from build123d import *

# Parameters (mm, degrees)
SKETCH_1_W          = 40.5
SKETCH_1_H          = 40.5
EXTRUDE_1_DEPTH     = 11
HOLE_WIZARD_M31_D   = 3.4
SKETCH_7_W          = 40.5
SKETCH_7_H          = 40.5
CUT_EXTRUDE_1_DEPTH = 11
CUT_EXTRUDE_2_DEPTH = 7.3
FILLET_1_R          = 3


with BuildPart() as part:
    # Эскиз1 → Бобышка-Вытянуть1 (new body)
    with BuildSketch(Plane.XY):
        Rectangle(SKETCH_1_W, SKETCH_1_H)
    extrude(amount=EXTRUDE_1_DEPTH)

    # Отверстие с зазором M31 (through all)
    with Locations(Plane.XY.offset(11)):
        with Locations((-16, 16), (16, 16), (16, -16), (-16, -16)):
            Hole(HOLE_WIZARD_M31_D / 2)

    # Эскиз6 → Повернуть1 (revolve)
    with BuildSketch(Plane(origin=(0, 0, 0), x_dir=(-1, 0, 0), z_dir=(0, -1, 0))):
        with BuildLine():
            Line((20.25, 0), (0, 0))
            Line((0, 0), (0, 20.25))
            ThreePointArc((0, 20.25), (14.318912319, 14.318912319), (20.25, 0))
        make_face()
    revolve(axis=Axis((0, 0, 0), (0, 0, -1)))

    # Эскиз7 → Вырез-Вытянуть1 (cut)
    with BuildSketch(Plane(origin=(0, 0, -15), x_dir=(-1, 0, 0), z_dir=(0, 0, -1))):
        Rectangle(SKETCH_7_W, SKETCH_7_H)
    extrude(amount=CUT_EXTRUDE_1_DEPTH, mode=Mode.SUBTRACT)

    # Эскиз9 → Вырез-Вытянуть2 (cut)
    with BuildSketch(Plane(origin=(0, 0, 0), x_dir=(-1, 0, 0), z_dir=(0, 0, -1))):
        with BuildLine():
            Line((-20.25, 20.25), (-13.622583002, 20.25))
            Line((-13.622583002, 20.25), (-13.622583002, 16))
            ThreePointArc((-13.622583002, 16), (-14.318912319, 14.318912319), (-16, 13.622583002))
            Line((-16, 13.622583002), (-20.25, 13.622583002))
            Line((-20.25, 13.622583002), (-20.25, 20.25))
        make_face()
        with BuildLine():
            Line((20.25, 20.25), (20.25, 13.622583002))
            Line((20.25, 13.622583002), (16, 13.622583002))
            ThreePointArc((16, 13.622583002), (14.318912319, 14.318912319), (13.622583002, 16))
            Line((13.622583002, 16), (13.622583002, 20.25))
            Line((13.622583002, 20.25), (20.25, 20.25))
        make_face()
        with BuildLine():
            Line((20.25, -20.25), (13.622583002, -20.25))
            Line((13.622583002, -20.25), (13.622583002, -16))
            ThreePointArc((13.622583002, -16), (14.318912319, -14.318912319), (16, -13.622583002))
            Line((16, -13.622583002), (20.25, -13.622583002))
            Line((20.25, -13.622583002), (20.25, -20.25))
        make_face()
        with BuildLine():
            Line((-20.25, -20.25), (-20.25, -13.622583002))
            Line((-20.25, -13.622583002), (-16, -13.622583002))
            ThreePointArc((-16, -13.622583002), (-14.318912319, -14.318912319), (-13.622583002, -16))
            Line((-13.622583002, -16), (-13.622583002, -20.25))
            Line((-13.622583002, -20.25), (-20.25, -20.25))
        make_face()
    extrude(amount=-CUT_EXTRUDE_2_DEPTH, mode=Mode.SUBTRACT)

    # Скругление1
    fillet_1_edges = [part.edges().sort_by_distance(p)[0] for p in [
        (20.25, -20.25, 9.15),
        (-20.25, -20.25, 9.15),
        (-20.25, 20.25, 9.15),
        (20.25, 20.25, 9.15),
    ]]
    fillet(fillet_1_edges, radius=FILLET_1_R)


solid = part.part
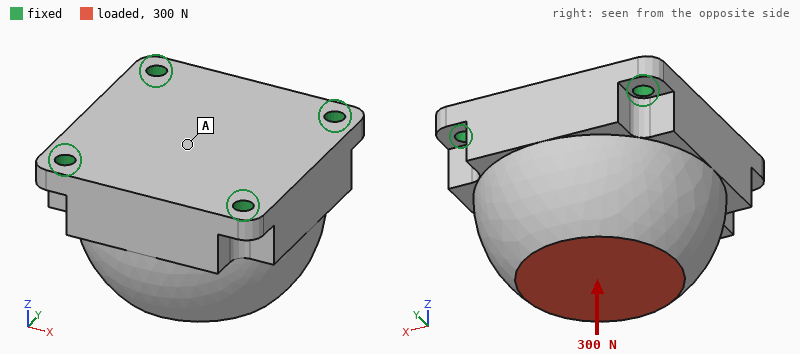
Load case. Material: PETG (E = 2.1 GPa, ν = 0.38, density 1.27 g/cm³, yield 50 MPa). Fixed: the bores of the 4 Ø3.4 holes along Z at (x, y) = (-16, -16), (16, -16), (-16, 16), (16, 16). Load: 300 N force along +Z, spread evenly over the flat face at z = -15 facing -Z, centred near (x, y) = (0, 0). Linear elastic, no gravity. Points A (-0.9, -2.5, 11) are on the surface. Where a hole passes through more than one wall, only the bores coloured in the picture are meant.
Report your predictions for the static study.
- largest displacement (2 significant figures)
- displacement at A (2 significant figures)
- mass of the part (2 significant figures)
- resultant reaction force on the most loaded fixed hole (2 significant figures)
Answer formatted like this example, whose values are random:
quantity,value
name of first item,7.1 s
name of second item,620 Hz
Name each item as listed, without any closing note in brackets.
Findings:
quantity,value
largest displacement,15 µm
displacement at A,12 µm
mass of the part,41 g
resultant reaction force on the most loaded fixed hole,83 N
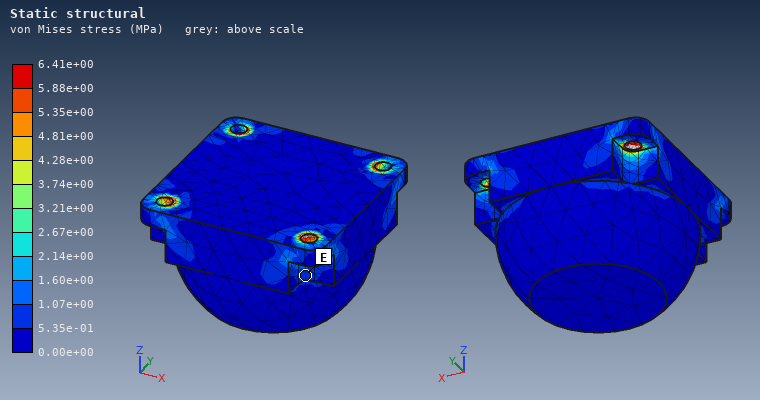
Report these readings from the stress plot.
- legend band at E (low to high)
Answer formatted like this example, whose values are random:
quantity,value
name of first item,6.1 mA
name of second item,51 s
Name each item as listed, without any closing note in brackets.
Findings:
quantity,value
legend band at E,5.35e-01 to 1.07e+00 MPa
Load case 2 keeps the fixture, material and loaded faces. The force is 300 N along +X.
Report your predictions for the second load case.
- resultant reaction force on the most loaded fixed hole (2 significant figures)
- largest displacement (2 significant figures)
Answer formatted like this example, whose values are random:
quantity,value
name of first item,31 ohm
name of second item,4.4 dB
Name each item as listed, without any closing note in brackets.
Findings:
quantity,value
resultant reaction force on the most loaded fixed hole,150 N
largest displacement,43 µm
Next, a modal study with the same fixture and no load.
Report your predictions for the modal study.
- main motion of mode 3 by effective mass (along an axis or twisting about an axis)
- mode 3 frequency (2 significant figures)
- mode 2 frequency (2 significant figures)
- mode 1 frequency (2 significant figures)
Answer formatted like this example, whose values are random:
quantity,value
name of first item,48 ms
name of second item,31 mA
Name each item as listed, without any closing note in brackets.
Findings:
quantity,value
main motion of mode 3 by effective mass,along Z
mode 3 frequency,4100 Hz
mode 2 frequency,3700 Hz
mode 1 frequency,3700 Hz
